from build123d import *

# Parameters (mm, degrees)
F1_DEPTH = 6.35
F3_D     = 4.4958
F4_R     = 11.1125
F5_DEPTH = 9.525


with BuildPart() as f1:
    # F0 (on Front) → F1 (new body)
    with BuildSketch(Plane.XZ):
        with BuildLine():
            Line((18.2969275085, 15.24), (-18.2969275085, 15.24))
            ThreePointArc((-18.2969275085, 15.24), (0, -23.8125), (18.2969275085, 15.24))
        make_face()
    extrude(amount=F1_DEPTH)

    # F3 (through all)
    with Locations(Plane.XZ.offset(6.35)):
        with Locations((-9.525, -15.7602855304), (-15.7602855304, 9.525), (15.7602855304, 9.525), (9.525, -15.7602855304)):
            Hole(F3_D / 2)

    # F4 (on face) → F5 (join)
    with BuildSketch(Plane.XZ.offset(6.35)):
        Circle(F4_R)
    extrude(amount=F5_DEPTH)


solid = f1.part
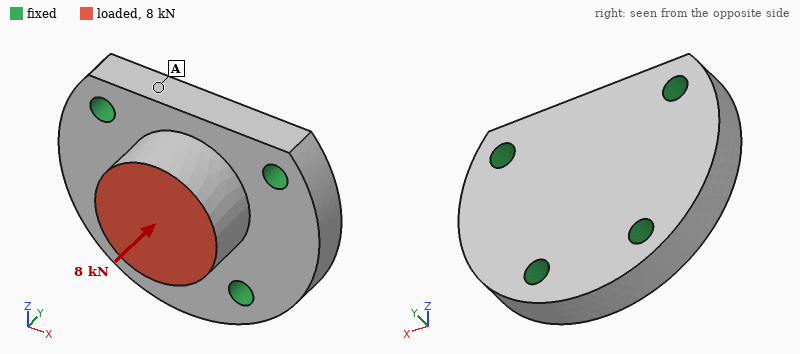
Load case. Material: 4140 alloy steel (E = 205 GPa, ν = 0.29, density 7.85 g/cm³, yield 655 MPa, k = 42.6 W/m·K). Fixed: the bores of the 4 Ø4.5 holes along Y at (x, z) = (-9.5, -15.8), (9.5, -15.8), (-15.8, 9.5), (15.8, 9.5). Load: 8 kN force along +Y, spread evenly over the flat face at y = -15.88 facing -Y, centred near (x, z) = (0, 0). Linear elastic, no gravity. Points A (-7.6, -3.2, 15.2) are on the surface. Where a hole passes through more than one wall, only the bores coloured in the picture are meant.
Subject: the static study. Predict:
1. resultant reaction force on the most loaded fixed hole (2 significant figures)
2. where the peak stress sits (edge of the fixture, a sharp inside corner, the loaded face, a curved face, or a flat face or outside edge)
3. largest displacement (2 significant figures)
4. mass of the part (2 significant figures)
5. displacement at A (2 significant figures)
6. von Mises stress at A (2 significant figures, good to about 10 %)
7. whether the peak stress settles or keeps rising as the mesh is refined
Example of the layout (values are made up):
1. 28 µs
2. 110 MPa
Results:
1. 2.5 kN
2. edge of the fixture
3. 7.6 µm
4. 100 g
5. 3.7 µm
6. 34 MPa
7. keeps rising
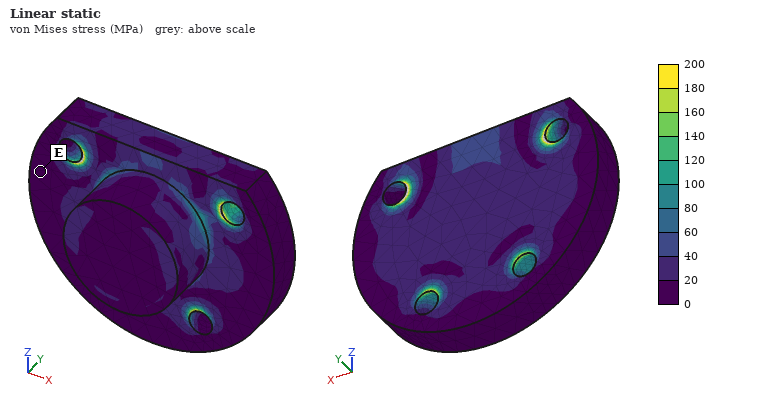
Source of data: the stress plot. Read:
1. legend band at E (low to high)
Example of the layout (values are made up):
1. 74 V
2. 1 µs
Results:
1. 0 to 20 MPa
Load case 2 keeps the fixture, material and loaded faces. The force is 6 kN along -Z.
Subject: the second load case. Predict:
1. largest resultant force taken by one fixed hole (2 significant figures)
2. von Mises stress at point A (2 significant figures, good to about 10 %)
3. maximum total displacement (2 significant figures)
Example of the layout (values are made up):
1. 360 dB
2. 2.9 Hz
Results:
1. 2.5 kN
2. 50 MPa
3. 13 µm
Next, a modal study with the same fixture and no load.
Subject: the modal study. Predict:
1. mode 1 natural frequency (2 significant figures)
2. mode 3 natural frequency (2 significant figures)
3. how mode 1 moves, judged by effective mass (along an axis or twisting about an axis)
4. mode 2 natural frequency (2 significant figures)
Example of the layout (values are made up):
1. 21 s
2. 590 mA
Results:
1. 24 kHz
2. 29 kHz
3. along Y
4. 28 kHz
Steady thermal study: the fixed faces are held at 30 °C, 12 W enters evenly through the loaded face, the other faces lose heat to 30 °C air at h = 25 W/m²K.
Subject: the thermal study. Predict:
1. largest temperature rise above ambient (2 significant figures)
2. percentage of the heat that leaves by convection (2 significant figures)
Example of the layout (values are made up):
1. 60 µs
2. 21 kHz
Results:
1. 15 K
2. 3.4 %
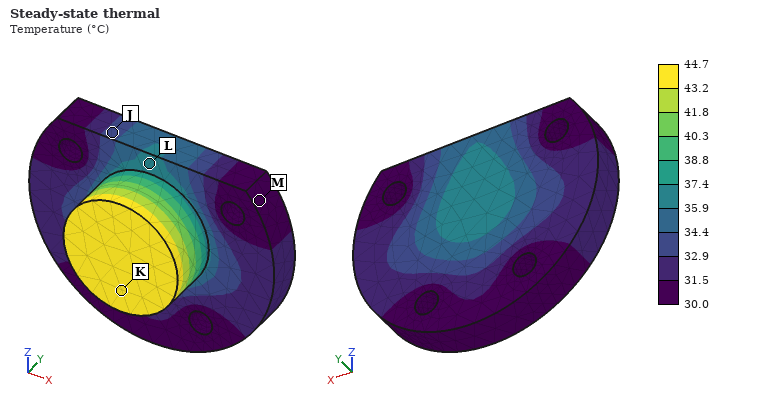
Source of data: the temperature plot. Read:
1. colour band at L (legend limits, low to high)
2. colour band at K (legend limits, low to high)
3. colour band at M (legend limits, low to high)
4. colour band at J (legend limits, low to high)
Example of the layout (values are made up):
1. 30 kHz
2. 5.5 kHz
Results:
1. 35.9 to 37.4 °C
2. 43.2 to 44.7 °C
3. 30.0 to 31.5 °C
4. 32.9 to 34.4 °C
